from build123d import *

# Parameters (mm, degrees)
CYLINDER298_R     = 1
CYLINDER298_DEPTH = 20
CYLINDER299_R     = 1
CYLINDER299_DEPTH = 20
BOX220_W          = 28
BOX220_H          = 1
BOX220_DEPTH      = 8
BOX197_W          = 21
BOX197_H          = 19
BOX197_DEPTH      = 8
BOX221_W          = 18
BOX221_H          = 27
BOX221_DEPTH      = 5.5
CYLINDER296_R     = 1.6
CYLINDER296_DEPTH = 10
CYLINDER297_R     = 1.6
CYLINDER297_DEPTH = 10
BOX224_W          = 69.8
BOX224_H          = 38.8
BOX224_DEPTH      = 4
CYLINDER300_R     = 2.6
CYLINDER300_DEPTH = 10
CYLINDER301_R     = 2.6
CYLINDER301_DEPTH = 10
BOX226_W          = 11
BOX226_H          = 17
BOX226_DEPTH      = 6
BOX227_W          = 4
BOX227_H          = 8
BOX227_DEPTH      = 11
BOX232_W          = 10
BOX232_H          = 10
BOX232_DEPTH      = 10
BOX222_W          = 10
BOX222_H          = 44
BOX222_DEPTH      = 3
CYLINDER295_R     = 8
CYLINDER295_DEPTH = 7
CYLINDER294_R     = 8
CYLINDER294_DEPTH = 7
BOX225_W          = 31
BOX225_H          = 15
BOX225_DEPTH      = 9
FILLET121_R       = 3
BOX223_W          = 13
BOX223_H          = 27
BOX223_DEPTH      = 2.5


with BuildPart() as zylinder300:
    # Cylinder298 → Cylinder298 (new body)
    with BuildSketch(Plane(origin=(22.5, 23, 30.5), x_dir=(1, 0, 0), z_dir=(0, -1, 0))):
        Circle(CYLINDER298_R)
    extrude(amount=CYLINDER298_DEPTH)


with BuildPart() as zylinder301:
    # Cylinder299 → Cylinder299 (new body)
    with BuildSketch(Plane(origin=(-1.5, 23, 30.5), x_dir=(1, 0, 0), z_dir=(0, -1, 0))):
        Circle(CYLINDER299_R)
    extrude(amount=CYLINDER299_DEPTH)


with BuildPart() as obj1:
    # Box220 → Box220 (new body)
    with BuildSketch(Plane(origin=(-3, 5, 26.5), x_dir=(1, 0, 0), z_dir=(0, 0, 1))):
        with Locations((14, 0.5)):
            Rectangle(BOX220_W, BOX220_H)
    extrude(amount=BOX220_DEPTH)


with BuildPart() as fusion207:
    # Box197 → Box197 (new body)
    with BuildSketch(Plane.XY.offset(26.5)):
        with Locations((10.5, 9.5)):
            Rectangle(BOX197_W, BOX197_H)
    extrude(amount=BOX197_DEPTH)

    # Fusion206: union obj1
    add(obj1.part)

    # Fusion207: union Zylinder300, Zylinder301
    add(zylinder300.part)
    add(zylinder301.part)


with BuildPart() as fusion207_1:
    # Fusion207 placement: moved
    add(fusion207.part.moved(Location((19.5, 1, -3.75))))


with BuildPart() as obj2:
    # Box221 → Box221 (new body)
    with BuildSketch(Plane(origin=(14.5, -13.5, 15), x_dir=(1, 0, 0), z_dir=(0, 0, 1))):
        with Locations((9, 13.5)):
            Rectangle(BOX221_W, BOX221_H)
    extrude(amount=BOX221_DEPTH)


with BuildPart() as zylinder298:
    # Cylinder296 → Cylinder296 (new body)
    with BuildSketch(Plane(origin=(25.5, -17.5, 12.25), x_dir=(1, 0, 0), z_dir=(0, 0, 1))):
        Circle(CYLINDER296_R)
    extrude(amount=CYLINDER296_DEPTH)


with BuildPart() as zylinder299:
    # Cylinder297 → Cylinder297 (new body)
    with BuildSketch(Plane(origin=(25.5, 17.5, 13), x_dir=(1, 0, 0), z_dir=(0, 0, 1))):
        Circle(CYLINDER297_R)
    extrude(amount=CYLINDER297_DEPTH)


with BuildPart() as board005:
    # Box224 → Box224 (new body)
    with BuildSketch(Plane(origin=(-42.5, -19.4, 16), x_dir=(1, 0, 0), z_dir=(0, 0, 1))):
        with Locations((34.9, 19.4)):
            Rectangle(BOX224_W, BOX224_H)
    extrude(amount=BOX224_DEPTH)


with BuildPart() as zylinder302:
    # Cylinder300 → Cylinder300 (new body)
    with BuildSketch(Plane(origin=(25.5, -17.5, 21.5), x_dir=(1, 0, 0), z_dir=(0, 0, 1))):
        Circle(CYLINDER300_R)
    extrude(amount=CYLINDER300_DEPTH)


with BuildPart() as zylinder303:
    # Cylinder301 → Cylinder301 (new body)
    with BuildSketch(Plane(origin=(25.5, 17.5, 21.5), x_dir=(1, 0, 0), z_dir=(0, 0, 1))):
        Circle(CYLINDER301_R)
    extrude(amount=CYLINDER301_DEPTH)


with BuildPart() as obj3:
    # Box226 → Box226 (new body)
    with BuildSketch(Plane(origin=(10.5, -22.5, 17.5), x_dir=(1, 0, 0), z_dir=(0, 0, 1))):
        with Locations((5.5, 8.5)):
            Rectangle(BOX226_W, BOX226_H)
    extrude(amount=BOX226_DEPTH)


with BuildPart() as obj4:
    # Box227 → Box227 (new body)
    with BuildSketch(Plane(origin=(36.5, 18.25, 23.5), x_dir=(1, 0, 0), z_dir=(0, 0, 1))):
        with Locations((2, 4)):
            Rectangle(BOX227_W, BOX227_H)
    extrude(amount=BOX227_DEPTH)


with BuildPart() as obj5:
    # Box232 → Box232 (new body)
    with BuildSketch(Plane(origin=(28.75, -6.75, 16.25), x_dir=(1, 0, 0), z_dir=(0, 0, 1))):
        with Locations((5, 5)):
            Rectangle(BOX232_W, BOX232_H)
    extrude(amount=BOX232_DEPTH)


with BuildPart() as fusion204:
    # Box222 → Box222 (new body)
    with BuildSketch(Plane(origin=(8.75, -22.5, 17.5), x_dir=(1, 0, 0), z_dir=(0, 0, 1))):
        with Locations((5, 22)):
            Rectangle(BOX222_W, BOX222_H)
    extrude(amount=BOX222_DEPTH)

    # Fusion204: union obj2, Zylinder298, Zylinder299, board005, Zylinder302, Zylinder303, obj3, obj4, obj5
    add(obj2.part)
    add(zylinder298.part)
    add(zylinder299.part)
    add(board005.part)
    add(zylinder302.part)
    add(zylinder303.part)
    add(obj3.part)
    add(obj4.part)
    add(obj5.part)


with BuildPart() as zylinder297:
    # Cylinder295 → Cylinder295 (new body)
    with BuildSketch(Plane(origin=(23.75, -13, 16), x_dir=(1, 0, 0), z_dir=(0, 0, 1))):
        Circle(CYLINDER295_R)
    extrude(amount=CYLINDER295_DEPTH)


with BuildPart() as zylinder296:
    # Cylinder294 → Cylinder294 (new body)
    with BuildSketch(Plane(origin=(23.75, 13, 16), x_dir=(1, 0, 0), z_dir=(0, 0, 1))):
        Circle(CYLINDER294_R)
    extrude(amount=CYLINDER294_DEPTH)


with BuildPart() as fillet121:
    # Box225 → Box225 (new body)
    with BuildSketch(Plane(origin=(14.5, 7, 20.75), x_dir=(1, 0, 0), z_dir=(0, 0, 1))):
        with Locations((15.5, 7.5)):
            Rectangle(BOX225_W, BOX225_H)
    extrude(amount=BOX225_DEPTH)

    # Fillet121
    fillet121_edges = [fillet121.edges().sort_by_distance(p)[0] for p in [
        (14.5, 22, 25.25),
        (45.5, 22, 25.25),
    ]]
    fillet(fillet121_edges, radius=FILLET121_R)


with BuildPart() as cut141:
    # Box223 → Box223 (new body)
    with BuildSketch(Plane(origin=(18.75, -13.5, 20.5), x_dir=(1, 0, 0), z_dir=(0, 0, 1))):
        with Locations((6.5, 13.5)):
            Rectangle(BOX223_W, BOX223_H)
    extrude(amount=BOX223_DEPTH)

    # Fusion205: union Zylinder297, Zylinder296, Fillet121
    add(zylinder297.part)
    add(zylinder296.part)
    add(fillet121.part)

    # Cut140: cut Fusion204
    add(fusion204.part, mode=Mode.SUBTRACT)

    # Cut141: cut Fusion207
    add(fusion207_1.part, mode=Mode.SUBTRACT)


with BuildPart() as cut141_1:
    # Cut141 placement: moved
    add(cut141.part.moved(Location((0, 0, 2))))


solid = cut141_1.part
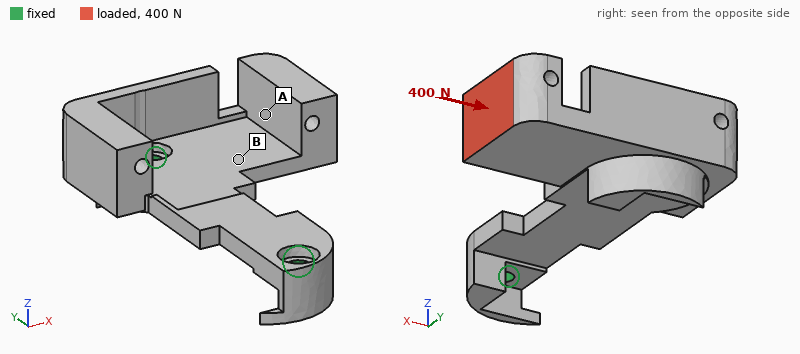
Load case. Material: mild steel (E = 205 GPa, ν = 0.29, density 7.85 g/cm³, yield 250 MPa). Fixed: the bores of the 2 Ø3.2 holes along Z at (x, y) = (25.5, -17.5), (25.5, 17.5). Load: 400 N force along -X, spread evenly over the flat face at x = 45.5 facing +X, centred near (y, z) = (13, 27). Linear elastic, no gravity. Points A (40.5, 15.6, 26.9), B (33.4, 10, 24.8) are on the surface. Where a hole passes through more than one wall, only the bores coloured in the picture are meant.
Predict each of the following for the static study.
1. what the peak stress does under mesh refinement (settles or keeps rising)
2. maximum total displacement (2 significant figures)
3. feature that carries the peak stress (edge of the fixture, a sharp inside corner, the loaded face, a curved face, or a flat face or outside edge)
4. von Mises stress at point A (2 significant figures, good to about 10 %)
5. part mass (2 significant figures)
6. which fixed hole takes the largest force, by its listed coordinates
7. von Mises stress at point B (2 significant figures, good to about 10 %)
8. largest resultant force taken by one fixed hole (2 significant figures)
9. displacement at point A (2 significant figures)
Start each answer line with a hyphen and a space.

- keeps rising
- 84 µm
- edge of the fixture
- 20 MPa
- 24 g
- (25.5, 17.5)
- 92 MPa
- 350 N
- 37 µm
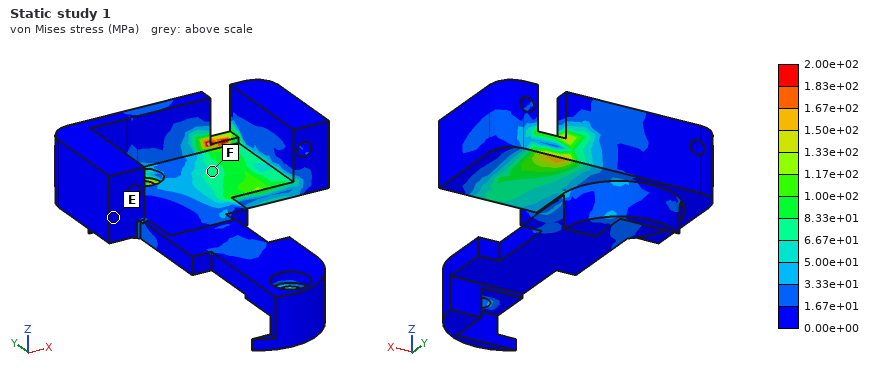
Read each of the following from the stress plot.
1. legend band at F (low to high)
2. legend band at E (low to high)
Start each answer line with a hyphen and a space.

- 6.67e+01 to 8.33e+01 MPa
- 0.00e+00 to 1.67e+01 MPa
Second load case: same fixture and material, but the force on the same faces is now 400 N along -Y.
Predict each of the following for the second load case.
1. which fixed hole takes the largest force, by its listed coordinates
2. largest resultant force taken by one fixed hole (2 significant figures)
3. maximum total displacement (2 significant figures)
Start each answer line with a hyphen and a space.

- (25.5, 17.5)
- 380 N
- 60 µm
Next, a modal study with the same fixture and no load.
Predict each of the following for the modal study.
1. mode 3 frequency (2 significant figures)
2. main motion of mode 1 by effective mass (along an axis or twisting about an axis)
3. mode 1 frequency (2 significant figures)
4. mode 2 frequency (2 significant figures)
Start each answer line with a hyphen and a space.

- 8900 Hz
- along Z
- 3200 Hz
- 6100 Hz
